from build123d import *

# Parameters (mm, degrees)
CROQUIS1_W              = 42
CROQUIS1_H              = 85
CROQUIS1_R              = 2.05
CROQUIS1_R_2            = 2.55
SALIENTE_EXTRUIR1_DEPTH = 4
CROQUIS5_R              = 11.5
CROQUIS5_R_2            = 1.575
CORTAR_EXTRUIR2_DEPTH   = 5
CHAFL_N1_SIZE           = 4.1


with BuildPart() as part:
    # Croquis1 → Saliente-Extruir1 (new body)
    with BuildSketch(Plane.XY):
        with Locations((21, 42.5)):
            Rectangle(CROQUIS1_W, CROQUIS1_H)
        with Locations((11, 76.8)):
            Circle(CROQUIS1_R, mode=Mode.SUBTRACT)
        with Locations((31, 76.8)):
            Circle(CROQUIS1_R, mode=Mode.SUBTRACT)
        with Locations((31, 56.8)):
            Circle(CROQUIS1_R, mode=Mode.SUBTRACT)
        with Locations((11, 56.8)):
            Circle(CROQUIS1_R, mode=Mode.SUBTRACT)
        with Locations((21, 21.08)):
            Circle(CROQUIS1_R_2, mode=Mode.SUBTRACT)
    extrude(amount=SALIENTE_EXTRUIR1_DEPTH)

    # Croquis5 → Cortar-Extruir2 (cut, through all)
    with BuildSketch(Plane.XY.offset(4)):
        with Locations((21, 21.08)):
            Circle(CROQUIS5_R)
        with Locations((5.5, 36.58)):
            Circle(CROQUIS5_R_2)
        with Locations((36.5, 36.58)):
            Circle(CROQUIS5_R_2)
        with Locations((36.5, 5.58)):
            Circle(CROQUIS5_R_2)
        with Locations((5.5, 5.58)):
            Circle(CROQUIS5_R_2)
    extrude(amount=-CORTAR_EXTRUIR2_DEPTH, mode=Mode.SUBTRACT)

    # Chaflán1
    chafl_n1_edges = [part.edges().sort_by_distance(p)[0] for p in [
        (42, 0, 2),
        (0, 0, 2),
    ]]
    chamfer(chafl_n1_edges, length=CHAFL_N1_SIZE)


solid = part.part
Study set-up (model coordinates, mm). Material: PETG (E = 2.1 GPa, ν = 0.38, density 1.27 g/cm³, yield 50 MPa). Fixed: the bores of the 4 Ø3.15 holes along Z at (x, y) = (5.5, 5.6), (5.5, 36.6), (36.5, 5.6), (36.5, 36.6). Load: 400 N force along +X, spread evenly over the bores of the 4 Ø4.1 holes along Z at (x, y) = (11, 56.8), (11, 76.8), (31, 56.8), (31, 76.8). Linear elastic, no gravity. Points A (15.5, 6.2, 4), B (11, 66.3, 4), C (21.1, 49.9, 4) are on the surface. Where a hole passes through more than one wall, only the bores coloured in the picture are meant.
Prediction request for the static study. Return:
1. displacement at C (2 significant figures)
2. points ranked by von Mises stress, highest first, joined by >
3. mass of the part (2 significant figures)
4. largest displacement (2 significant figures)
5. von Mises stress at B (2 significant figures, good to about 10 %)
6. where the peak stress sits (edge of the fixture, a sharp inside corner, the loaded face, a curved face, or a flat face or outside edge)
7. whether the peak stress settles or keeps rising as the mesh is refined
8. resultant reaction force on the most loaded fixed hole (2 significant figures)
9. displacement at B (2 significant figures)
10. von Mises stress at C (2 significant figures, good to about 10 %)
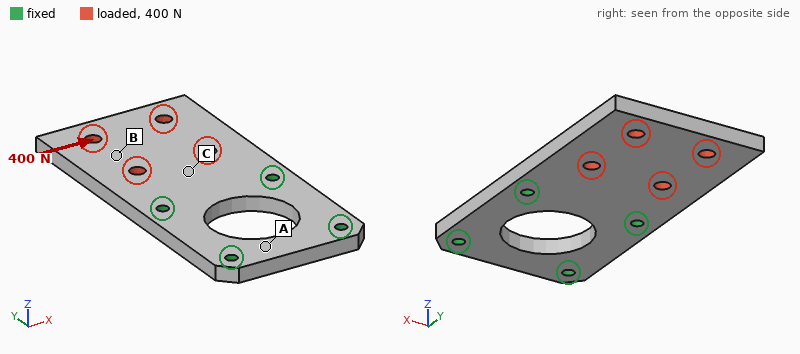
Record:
0.073 mm
C > B > A
16 g
0.30 mm
3.0 MPa
edge of the fixture
keeps rising
400 N
0.19 mm
5.5 MPa
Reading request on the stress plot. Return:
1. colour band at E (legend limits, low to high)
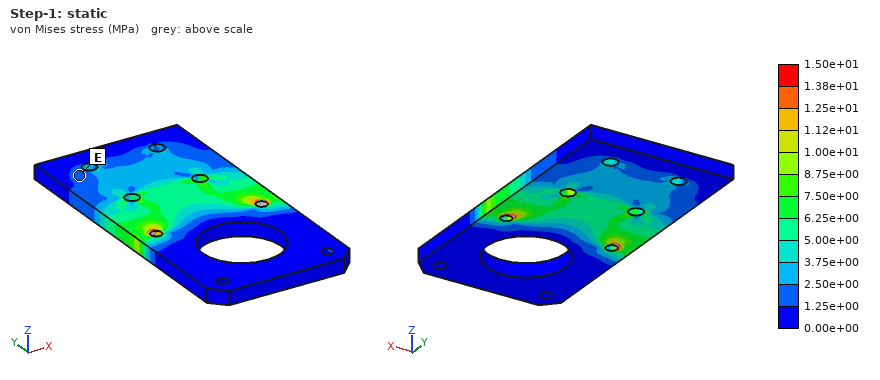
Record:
1.25e+00 to 2.50e+00 MPa
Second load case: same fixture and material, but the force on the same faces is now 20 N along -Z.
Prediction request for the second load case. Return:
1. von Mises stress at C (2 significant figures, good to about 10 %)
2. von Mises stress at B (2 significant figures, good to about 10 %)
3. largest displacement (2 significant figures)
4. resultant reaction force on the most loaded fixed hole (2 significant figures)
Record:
2.7 MPa
1.1 MPa
0.91 mm
12 N
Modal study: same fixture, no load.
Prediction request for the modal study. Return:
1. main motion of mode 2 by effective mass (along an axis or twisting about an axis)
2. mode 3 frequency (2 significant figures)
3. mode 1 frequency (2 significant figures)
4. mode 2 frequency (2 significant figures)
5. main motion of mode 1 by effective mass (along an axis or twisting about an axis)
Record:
twisting about Y
2000 Hz
340 Hz
930 Hz
along Z
